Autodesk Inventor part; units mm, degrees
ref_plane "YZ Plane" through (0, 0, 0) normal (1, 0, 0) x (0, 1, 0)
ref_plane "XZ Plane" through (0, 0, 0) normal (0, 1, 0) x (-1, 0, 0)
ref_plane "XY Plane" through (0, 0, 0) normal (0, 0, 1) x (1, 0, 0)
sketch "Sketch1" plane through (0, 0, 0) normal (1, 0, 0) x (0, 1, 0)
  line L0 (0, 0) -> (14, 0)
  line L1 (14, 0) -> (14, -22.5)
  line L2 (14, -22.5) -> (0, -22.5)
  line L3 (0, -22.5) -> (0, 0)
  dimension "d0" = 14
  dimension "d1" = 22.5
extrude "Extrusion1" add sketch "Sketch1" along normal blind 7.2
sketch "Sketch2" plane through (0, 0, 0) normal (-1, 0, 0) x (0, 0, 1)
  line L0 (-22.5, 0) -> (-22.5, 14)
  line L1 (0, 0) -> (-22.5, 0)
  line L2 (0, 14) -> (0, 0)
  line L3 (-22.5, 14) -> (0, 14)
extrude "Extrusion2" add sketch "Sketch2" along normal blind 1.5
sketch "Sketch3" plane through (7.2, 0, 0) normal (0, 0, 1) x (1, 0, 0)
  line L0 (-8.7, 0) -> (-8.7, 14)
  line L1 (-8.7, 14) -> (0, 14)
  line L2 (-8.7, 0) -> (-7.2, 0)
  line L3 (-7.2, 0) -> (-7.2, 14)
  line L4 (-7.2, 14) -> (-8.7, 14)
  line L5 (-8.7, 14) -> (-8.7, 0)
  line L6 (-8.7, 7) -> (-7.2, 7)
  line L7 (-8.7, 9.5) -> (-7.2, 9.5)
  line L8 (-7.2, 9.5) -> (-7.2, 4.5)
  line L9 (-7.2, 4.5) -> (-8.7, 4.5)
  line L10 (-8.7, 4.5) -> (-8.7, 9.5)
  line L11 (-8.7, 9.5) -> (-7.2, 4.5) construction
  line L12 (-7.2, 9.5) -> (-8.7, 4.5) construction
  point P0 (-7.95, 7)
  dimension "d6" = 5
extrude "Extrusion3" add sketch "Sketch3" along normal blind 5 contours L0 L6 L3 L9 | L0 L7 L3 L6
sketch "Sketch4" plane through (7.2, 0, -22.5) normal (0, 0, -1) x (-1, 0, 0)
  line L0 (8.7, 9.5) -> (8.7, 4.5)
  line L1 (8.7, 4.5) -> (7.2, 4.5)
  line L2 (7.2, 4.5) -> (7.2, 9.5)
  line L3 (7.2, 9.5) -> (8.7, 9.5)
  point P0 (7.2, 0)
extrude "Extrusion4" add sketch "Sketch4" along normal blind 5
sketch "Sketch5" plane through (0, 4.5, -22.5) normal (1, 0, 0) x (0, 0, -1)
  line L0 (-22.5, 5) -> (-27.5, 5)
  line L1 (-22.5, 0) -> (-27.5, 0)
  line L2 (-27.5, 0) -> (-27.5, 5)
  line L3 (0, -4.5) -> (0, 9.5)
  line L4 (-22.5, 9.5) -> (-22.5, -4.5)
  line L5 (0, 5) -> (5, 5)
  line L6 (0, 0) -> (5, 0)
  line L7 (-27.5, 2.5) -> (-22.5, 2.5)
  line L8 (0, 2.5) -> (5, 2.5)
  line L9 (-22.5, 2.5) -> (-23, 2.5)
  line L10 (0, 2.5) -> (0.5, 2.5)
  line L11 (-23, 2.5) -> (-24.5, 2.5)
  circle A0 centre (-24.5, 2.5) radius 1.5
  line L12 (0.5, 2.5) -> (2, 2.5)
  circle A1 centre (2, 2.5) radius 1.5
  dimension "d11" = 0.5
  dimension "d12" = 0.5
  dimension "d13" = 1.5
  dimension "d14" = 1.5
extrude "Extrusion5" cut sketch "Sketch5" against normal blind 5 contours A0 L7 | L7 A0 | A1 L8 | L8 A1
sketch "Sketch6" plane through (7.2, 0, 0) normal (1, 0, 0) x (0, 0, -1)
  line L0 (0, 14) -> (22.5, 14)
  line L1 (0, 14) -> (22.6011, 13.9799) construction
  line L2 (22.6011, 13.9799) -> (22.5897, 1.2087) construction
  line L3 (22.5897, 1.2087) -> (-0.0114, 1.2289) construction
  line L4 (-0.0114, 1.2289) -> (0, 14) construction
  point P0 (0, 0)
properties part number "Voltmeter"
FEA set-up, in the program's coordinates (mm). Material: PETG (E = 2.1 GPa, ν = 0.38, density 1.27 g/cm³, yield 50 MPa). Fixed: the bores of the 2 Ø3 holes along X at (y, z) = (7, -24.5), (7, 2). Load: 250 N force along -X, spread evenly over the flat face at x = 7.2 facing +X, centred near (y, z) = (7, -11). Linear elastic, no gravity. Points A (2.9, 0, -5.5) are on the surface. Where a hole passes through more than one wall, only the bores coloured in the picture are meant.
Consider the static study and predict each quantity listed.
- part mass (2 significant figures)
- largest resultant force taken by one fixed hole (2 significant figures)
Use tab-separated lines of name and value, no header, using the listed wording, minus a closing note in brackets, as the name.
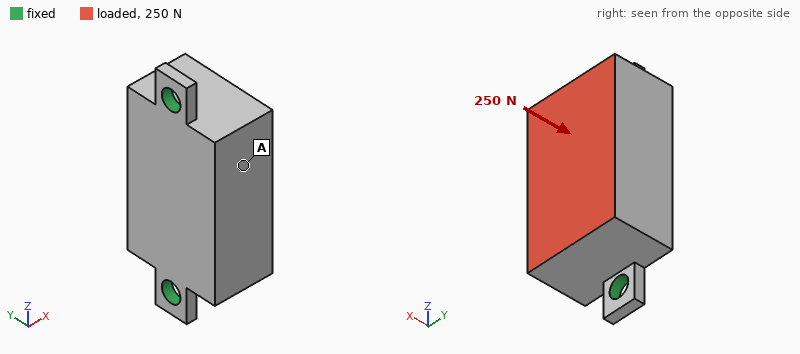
part mass	3.5 g
largest resultant force taken by one fixed hole	150 N
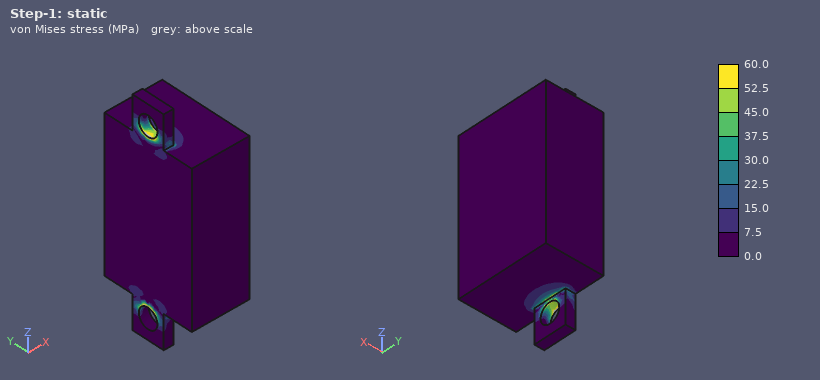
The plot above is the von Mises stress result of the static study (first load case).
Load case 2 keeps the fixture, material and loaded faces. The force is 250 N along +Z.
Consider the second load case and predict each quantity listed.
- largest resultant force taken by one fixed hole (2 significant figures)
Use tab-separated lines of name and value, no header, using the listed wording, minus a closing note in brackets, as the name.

largest resultant force taken by one fixed hole	150 N
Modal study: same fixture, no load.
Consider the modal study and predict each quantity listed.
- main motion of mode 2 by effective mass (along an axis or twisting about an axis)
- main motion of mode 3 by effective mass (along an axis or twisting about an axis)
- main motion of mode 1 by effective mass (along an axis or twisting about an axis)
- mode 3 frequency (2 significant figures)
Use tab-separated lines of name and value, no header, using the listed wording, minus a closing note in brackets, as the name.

main motion of mode 2 by effective mass	along X
main motion of mode 3 by effective mass	along Y
main motion of mode 1 by effective mass	along Y
mode 3 frequency	7100 Hz
